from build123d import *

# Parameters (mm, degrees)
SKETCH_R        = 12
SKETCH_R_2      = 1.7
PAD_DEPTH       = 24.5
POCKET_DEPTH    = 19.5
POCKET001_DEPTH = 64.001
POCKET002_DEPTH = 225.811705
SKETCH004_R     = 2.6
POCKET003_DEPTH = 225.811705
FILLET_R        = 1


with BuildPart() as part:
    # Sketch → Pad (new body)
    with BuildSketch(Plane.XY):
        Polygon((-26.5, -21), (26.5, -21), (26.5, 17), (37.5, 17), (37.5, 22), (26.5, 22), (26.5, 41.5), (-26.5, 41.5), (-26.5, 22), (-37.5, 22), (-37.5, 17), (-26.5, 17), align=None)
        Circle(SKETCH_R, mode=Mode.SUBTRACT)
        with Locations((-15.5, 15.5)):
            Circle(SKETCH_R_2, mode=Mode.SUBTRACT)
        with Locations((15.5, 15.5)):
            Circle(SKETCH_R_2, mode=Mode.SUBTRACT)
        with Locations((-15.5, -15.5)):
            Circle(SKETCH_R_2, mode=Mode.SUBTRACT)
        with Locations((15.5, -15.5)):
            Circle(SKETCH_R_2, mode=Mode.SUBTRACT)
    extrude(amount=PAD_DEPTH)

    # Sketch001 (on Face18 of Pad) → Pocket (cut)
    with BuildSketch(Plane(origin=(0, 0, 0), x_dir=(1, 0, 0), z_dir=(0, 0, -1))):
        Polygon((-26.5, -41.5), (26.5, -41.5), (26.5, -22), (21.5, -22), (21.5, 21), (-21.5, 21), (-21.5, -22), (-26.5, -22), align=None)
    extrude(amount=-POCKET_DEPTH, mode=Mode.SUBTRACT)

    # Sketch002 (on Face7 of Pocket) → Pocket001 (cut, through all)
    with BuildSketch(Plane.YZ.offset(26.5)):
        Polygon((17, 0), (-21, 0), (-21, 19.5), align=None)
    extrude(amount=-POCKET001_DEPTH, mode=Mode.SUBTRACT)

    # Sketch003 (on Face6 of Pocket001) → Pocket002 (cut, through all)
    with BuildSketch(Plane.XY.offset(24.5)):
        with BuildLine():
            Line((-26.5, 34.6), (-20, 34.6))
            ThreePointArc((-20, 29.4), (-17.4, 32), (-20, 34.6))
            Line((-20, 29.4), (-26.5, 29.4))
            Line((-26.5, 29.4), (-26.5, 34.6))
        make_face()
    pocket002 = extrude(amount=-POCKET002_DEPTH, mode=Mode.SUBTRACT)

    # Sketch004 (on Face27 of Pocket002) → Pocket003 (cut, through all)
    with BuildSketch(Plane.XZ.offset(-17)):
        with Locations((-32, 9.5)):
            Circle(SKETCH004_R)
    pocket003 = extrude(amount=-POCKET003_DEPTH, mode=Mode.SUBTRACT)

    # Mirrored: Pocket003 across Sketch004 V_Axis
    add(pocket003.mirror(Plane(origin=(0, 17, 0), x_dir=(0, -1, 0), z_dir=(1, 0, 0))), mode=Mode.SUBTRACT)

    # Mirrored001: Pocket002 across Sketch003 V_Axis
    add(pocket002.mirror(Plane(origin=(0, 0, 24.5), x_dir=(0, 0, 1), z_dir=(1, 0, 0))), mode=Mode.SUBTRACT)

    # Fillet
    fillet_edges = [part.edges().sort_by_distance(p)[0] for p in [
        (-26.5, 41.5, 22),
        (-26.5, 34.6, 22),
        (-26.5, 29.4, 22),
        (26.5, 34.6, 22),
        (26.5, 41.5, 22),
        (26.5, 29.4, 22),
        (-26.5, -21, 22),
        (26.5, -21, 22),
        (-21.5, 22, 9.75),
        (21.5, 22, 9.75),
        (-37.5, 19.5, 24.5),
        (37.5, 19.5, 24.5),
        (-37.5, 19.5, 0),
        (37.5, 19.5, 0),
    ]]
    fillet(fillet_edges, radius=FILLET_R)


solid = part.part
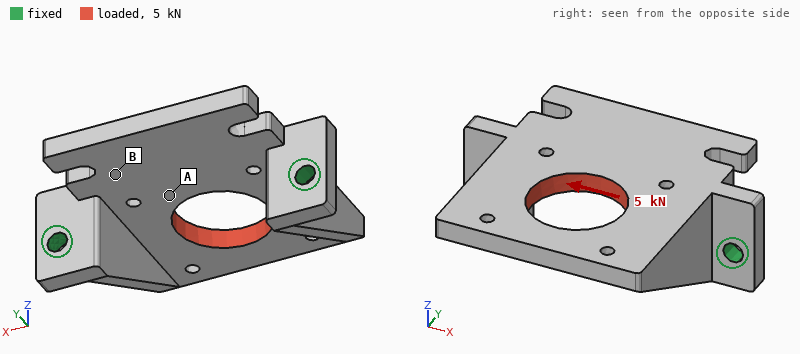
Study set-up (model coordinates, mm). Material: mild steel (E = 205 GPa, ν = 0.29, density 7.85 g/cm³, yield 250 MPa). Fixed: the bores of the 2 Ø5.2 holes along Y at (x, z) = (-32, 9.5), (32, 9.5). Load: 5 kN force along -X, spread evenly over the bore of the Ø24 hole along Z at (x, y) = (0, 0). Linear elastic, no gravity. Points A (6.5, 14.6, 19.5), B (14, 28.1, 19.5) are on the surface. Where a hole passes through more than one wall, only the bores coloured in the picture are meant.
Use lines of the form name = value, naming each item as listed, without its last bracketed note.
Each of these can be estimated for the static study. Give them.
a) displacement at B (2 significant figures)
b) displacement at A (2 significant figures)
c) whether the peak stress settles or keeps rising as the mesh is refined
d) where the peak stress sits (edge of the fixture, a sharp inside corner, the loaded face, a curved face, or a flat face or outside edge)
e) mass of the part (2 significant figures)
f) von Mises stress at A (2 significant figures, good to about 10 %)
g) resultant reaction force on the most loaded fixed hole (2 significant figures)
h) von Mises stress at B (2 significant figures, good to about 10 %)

displacement at B = 10 µm
displacement at A = 18 µm
whether the peak stress settles or keeps rising as the mesh is refined = keeps rising
where the peak stress sits = edge of the fixture
mass of the part = 160 g
von Mises stress at A = 70 MPa
resultant reaction force on the most loaded fixed hole = 3.0 kN
von Mises stress at B = 33 MPa
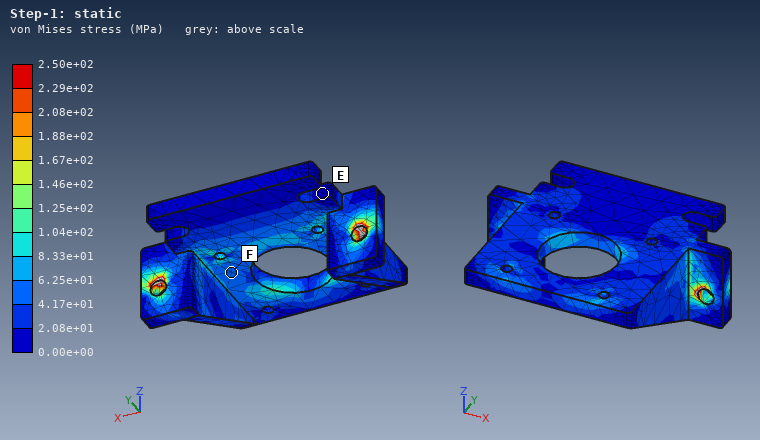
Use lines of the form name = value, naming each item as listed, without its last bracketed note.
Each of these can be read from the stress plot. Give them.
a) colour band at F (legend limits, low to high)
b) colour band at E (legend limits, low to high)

colour band at F = 4.17e+01 to 6.25e+01 MPa
colour band at E = 0.00e+00 to 2.08e+01 MPa
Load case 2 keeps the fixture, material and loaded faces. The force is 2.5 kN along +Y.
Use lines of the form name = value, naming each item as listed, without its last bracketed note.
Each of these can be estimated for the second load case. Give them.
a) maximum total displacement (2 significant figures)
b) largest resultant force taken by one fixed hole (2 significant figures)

maximum total displacement = 61 µm
largest resultant force taken by one fixed hole = 1.3 kN
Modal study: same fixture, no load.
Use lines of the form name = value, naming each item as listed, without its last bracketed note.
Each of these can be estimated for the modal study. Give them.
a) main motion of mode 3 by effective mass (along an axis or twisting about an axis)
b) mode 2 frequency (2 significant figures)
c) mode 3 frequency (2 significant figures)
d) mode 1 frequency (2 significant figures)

main motion of mode 3 by effective mass = along Z
mode 2 frequency = 4500 Hz
mode 3 frequency = 4800 Hz
mode 1 frequency = 2600 Hz
